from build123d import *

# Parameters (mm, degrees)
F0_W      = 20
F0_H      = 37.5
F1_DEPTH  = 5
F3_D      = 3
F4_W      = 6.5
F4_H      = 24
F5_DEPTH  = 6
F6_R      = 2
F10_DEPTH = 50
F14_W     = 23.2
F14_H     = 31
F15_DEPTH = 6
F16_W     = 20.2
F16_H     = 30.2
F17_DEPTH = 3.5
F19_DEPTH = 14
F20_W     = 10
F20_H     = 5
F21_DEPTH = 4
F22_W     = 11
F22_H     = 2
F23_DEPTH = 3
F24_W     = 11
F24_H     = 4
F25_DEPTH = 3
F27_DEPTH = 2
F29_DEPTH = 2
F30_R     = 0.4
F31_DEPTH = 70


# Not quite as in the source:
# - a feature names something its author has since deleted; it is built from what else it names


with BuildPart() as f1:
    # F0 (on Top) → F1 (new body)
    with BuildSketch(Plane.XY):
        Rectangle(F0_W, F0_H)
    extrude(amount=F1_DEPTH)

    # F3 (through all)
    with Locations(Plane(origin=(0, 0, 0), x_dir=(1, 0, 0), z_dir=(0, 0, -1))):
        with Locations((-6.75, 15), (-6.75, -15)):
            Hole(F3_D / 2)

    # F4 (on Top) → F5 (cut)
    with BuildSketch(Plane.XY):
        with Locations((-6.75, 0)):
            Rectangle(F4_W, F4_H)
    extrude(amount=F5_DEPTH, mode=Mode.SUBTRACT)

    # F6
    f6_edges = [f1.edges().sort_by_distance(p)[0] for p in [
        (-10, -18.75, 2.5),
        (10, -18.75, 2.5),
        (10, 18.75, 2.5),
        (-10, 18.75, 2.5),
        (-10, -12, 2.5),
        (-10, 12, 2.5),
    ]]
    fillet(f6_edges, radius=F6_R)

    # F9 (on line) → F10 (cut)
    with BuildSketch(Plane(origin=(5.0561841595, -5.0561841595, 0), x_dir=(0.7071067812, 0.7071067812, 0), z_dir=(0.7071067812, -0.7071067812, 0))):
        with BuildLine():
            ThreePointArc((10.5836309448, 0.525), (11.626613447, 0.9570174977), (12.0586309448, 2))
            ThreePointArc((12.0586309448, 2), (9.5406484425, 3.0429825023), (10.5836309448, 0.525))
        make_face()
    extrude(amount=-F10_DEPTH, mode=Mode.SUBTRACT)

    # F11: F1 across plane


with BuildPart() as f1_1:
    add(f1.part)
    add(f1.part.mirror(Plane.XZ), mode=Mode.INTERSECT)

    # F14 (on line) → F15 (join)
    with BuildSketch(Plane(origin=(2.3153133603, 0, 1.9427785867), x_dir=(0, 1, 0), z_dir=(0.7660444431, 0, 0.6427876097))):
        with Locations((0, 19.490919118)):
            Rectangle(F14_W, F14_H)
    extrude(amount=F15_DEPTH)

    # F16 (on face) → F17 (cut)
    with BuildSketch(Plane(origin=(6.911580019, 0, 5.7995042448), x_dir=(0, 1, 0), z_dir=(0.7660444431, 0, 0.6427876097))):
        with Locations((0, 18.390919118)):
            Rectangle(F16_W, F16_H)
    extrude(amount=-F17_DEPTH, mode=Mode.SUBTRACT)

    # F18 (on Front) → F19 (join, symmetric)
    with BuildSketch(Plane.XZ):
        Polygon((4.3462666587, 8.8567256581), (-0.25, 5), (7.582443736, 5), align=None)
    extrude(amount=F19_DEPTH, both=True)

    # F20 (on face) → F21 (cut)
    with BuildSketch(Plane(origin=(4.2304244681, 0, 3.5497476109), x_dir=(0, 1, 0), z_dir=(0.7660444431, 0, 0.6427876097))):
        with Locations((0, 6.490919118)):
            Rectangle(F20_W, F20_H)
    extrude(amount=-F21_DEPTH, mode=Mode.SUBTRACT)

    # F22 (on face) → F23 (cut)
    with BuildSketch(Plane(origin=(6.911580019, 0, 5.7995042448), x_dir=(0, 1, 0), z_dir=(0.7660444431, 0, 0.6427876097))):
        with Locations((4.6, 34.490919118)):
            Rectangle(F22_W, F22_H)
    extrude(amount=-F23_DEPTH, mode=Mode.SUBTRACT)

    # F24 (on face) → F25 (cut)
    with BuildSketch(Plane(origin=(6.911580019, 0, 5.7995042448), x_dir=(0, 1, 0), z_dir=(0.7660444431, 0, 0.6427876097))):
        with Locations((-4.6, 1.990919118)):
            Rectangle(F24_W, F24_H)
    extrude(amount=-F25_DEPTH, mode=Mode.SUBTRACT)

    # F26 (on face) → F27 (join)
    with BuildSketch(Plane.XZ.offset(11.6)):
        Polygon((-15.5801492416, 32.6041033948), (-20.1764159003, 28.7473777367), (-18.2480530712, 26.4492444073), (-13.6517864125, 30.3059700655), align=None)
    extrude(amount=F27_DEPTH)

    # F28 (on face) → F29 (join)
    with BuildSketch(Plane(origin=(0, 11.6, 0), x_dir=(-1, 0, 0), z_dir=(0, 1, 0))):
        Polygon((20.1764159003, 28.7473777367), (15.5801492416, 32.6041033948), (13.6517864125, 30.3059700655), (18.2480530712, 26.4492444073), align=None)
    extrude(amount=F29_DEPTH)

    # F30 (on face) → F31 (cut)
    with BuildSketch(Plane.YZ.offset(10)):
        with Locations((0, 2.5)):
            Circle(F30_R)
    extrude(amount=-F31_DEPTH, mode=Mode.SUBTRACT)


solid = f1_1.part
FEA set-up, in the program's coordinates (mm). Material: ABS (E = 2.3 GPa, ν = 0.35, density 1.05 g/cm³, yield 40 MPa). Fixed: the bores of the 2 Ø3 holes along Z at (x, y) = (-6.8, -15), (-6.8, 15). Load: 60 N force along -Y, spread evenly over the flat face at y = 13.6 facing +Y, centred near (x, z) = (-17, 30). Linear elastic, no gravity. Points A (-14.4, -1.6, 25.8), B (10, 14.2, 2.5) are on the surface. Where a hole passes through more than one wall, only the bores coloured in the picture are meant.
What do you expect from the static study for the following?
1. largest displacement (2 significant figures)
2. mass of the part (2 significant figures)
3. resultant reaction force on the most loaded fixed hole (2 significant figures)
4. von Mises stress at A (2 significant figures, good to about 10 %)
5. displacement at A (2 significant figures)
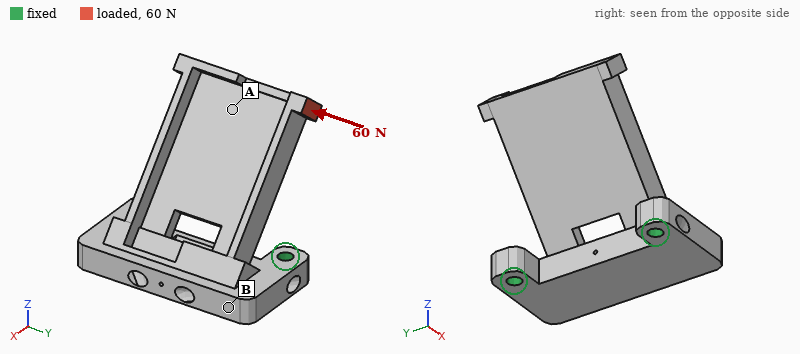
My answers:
0.67 mm
5.3 g
69 N
5.1 MPa
0.27 mm
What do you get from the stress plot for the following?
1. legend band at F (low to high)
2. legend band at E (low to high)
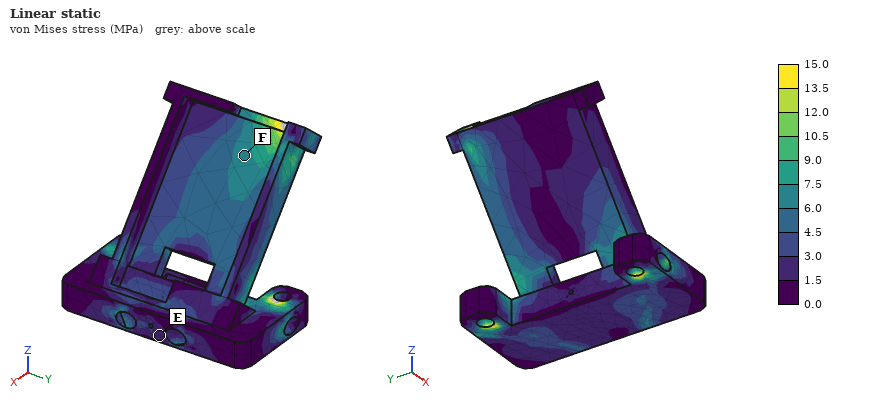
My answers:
6.0 to 7.5 MPa
1.5 to 3.0 MPa
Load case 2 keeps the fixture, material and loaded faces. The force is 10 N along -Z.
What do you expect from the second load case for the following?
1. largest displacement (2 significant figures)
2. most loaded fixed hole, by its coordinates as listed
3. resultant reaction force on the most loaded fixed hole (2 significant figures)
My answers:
0.64 mm
(-6.8, 15)
10 N
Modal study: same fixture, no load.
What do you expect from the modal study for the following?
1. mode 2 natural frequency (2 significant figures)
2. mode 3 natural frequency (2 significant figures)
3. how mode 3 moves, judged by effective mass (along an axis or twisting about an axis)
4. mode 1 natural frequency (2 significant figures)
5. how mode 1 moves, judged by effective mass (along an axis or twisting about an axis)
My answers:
1500 Hz
2100 Hz
along Y
640 Hz
along X
